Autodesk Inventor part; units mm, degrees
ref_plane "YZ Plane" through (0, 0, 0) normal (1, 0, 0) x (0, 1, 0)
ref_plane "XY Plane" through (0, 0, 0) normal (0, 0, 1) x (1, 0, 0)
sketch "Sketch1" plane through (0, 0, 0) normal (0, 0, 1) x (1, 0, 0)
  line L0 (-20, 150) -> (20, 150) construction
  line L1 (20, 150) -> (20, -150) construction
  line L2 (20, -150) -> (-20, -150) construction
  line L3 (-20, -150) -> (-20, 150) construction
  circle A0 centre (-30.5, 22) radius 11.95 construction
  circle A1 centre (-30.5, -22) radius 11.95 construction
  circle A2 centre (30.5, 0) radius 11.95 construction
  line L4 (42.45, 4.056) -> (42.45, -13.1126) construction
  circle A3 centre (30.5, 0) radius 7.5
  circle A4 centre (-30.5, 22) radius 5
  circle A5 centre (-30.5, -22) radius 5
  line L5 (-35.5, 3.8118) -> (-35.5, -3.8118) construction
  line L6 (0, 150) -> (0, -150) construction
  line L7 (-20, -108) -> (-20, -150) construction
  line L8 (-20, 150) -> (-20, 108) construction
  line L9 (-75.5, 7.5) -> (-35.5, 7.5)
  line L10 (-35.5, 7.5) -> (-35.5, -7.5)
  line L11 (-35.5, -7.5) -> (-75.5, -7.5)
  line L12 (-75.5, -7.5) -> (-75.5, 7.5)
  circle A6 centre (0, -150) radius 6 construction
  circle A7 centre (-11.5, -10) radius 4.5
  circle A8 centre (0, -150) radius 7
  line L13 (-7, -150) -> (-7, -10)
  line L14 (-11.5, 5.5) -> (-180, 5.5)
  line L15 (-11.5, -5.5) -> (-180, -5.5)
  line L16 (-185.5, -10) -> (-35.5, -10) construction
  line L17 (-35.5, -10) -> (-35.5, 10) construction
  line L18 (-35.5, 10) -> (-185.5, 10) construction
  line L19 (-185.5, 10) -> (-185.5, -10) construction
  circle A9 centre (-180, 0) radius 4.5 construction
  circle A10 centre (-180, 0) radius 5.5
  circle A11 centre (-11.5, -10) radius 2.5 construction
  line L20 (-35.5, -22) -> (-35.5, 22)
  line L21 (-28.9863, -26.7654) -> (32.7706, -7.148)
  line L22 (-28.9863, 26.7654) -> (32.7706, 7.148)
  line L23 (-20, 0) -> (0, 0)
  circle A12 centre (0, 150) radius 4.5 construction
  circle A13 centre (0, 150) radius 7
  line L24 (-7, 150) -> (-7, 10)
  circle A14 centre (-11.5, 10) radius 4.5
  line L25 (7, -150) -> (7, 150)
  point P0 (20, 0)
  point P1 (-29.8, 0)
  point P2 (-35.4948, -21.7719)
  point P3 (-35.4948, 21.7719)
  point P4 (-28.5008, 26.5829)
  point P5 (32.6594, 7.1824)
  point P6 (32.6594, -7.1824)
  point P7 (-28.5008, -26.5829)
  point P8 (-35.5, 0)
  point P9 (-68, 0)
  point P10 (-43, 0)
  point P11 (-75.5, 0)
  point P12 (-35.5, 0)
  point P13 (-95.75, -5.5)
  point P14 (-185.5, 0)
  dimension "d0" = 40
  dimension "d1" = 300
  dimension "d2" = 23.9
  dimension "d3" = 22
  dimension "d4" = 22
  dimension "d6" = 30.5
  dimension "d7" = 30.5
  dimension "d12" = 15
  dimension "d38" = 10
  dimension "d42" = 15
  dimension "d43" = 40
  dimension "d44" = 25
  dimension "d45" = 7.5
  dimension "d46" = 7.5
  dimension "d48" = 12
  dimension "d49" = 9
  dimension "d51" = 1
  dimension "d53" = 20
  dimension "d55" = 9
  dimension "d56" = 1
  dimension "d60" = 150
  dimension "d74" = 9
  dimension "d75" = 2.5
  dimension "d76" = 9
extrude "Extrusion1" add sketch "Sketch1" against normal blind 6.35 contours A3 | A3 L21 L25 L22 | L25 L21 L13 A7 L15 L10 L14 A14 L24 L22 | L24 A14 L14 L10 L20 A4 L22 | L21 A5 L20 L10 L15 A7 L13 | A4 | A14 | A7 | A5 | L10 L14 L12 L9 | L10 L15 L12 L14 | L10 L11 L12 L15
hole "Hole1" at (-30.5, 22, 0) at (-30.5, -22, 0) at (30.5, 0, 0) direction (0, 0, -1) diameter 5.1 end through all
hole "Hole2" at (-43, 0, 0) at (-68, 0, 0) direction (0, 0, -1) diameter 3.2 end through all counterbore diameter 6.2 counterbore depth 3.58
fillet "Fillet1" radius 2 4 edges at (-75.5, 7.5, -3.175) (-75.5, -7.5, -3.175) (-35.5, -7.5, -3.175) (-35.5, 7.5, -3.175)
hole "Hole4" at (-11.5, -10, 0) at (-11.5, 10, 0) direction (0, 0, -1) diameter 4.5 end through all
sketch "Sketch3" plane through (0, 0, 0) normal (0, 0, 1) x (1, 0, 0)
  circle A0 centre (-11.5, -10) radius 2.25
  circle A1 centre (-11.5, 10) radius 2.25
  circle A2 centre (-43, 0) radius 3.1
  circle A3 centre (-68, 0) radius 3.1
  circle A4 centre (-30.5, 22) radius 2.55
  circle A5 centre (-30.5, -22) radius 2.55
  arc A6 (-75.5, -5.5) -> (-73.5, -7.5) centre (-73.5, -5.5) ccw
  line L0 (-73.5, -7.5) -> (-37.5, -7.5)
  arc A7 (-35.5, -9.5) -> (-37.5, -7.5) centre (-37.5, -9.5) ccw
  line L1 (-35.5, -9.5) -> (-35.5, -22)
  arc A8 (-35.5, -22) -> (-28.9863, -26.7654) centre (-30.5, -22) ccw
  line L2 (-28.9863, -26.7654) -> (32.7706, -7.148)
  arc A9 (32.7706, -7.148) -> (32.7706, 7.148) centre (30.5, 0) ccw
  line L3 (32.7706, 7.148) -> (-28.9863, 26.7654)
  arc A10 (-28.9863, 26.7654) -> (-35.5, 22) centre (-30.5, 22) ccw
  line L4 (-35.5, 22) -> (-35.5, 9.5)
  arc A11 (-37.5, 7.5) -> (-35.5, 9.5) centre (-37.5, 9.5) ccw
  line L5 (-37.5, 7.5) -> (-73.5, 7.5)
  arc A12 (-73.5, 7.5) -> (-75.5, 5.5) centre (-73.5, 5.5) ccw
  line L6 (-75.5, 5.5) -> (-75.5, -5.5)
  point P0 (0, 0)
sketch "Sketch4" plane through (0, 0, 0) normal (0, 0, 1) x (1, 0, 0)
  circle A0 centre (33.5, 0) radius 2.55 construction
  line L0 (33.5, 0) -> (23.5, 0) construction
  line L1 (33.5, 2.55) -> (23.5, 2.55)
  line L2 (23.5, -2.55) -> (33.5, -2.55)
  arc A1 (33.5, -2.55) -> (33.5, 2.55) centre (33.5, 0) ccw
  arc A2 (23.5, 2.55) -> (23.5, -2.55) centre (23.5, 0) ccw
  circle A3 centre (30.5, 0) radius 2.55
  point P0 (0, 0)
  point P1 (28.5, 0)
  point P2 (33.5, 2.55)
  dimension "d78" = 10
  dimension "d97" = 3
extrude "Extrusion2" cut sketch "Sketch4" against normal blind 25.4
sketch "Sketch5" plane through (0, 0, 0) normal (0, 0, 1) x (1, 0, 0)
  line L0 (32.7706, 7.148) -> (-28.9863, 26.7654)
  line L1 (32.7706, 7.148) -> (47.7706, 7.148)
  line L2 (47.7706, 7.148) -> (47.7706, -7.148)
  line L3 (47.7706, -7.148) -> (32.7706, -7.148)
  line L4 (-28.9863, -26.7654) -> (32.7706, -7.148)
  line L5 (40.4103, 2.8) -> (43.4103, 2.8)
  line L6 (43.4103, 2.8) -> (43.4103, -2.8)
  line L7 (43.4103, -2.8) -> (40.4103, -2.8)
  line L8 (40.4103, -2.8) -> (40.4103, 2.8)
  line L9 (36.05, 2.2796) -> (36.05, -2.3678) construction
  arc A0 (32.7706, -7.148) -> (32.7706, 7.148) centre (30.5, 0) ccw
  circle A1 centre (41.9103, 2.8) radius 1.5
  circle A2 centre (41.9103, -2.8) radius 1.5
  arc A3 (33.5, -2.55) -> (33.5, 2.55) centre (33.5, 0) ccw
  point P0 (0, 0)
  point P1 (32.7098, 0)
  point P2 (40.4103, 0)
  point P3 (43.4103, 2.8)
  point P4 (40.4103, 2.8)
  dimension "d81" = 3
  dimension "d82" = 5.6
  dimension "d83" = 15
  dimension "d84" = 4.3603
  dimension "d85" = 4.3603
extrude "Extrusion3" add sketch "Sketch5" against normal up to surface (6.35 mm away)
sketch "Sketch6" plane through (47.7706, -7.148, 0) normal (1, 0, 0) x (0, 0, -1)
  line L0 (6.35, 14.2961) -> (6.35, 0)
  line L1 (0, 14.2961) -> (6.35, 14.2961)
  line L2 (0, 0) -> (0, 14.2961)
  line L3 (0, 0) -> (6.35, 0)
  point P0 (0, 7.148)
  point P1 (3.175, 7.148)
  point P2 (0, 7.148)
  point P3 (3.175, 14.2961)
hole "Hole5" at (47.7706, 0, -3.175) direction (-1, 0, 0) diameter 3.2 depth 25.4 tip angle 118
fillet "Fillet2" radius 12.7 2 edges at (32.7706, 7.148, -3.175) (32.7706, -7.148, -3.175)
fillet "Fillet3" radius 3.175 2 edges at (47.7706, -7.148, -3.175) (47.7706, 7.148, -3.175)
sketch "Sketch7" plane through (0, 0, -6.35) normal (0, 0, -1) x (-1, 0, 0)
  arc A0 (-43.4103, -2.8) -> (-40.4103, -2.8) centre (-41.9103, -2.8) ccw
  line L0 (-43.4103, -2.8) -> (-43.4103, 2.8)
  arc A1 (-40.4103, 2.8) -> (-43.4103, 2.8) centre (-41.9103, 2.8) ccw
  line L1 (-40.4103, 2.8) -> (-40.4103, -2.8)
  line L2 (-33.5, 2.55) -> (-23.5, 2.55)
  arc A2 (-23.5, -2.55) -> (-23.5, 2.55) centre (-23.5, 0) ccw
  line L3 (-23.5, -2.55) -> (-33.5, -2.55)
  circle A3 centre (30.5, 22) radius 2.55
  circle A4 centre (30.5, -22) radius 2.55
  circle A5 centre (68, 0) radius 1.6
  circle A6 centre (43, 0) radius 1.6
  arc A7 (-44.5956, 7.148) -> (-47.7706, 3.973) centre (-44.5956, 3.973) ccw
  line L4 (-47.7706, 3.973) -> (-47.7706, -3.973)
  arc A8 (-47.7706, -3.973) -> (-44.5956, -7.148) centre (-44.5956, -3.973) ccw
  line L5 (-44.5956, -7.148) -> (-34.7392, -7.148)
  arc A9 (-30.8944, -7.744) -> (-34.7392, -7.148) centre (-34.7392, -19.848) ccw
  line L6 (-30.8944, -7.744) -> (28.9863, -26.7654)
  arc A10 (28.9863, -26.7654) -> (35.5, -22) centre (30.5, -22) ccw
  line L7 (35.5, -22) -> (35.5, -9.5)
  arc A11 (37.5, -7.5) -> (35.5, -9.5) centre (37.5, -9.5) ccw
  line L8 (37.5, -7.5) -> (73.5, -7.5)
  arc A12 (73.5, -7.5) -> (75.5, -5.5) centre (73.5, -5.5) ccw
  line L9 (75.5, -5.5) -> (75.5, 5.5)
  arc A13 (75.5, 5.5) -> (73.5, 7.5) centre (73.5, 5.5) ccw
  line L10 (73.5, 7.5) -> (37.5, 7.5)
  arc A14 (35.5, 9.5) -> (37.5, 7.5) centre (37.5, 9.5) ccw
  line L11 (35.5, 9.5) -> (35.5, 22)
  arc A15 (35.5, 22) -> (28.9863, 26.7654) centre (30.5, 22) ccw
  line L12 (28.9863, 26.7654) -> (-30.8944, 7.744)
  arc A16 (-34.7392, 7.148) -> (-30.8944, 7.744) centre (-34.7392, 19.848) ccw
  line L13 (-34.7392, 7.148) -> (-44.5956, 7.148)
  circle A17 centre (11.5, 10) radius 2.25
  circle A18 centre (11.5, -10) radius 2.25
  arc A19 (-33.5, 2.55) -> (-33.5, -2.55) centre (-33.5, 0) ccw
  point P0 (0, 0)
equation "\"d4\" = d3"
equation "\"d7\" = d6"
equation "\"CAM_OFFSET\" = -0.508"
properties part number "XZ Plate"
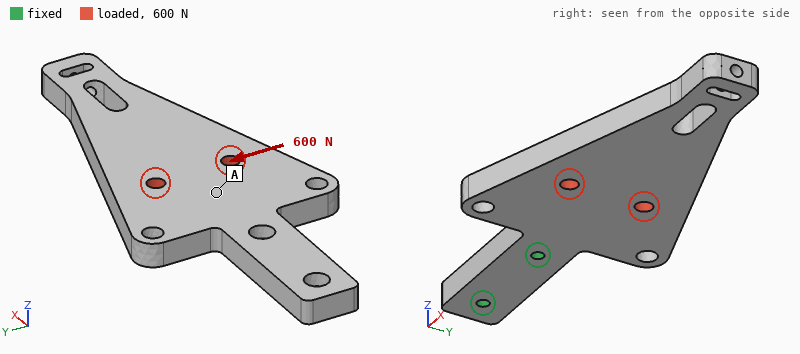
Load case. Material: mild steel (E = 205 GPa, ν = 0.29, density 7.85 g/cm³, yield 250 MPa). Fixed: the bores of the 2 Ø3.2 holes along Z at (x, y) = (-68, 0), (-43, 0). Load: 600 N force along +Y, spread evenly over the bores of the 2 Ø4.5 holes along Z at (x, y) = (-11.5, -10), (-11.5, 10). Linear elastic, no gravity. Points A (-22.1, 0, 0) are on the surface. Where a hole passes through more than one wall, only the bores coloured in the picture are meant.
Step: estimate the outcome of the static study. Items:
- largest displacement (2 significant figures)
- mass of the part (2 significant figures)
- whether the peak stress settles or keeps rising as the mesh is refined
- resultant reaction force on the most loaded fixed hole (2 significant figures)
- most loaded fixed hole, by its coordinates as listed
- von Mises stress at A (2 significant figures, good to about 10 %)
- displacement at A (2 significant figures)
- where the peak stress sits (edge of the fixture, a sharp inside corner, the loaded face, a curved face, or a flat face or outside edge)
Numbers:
93 µm
150 g
keeps rising
1.2 kN
(-43, 0)
11 MPa
21 µm
edge of the fixture
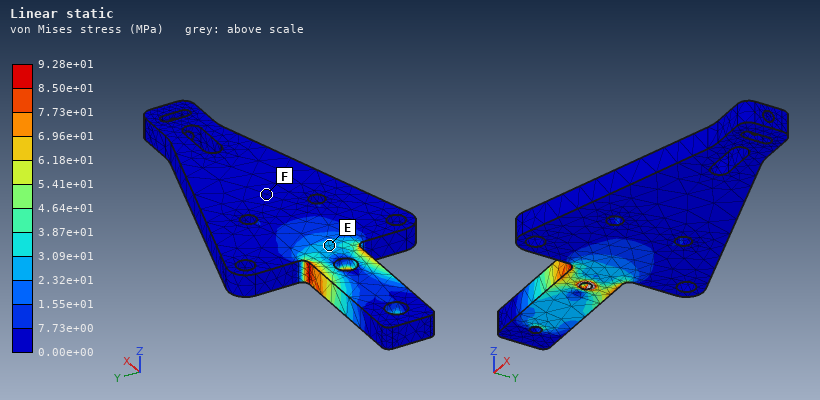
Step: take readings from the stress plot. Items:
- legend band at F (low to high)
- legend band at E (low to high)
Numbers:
0.00e+00 to 7.73e+00 MPa
2.32e+01 to 3.09e+01 MPa
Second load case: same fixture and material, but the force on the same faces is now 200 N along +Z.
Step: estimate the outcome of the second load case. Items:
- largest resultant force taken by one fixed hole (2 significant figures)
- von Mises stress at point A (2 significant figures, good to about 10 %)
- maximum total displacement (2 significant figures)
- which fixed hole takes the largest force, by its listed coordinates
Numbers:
570 N
8.5 MPa
0.14 mm
(-43, 0)
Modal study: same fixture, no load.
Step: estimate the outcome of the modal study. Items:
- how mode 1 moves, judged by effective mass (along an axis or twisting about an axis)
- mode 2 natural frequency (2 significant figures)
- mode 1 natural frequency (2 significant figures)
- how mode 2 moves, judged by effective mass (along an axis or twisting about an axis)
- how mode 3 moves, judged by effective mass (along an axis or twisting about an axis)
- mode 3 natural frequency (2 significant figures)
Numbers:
along Z
1400 Hz
630 Hz
along Y
twisting about X
2100 Hz
